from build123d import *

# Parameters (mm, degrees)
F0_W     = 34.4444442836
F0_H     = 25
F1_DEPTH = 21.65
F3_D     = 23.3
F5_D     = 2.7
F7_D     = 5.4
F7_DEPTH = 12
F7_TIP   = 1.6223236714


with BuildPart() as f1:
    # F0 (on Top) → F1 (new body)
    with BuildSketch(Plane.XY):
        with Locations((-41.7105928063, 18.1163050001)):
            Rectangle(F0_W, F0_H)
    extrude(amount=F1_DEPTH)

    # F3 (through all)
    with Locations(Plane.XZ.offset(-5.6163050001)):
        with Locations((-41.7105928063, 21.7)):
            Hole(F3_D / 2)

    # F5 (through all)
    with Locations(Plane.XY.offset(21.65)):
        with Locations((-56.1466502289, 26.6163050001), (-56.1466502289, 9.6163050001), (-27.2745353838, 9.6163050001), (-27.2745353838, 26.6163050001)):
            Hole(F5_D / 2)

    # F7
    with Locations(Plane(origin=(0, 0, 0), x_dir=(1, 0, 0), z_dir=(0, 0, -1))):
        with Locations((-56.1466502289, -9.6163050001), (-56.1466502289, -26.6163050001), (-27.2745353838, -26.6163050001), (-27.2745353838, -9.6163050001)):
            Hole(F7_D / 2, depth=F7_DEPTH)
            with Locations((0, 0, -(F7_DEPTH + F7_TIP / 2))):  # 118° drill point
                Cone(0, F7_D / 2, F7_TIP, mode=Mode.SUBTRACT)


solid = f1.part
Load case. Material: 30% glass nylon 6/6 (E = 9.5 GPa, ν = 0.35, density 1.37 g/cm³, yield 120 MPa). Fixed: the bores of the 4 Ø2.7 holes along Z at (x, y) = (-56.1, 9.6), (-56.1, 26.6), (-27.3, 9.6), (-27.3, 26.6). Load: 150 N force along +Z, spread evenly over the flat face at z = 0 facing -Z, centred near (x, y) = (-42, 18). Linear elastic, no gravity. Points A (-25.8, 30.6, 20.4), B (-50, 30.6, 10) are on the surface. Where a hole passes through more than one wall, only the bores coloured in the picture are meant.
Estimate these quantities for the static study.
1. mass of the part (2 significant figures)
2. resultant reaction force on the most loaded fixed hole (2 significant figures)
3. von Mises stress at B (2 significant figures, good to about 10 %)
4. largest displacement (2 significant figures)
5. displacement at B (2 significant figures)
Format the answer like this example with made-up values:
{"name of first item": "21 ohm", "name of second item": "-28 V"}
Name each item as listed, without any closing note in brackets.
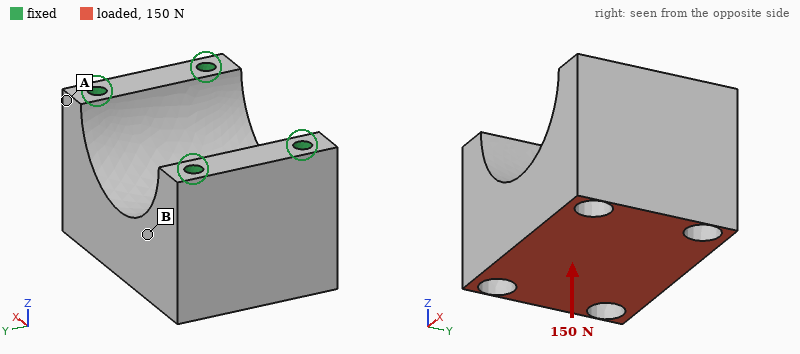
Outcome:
{"mass of the part": "16 g", "resultant reaction force on the most loaded fixed hole": "42 N", "von Mises stress at B": "0.42 MPa", "largest displacement": "1.2 µm", "displacement at B": "0.73 µm"}
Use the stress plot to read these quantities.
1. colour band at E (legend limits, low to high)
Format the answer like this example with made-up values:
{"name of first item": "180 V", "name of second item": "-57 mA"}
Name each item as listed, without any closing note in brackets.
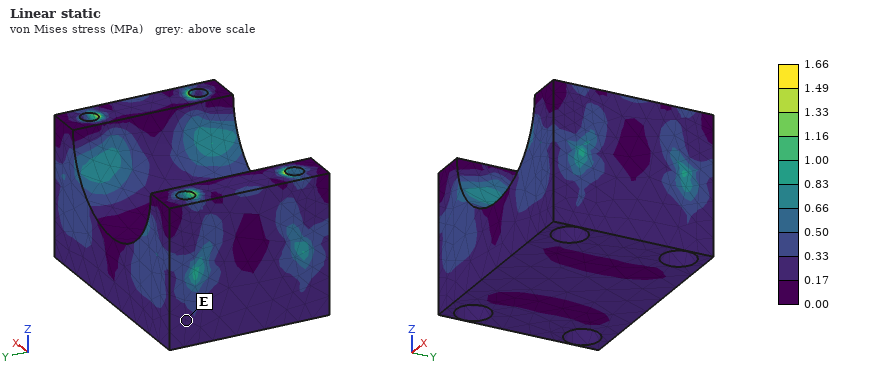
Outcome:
{"colour band at E": "0.17 to 0.33 MPa"}
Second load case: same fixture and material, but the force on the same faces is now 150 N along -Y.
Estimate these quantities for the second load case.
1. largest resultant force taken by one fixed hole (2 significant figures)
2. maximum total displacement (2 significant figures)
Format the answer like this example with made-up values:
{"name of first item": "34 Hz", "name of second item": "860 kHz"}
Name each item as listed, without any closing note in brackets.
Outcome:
{"largest resultant force taken by one fixed hole": "76 N", "maximum total displacement": "4.7 µm"}
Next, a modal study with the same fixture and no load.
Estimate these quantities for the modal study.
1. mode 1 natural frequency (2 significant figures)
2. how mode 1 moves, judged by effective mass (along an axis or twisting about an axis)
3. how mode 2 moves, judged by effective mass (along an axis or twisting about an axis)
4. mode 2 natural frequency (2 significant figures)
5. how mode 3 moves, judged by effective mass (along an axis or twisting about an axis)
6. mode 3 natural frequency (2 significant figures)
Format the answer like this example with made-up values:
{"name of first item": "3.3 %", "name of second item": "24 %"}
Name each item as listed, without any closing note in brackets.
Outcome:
{"mode 1 natural frequency": "12 kHz", "how mode 1 moves, judged by effective mass": "along Y", "how mode 2 moves, judged by effective mass": "along X", "mode 2 natural frequency": "15 kHz", "how mode 3 moves, judged by effective mass": "twisting about Z", "mode 3 natural frequency": "18 kHz"}
